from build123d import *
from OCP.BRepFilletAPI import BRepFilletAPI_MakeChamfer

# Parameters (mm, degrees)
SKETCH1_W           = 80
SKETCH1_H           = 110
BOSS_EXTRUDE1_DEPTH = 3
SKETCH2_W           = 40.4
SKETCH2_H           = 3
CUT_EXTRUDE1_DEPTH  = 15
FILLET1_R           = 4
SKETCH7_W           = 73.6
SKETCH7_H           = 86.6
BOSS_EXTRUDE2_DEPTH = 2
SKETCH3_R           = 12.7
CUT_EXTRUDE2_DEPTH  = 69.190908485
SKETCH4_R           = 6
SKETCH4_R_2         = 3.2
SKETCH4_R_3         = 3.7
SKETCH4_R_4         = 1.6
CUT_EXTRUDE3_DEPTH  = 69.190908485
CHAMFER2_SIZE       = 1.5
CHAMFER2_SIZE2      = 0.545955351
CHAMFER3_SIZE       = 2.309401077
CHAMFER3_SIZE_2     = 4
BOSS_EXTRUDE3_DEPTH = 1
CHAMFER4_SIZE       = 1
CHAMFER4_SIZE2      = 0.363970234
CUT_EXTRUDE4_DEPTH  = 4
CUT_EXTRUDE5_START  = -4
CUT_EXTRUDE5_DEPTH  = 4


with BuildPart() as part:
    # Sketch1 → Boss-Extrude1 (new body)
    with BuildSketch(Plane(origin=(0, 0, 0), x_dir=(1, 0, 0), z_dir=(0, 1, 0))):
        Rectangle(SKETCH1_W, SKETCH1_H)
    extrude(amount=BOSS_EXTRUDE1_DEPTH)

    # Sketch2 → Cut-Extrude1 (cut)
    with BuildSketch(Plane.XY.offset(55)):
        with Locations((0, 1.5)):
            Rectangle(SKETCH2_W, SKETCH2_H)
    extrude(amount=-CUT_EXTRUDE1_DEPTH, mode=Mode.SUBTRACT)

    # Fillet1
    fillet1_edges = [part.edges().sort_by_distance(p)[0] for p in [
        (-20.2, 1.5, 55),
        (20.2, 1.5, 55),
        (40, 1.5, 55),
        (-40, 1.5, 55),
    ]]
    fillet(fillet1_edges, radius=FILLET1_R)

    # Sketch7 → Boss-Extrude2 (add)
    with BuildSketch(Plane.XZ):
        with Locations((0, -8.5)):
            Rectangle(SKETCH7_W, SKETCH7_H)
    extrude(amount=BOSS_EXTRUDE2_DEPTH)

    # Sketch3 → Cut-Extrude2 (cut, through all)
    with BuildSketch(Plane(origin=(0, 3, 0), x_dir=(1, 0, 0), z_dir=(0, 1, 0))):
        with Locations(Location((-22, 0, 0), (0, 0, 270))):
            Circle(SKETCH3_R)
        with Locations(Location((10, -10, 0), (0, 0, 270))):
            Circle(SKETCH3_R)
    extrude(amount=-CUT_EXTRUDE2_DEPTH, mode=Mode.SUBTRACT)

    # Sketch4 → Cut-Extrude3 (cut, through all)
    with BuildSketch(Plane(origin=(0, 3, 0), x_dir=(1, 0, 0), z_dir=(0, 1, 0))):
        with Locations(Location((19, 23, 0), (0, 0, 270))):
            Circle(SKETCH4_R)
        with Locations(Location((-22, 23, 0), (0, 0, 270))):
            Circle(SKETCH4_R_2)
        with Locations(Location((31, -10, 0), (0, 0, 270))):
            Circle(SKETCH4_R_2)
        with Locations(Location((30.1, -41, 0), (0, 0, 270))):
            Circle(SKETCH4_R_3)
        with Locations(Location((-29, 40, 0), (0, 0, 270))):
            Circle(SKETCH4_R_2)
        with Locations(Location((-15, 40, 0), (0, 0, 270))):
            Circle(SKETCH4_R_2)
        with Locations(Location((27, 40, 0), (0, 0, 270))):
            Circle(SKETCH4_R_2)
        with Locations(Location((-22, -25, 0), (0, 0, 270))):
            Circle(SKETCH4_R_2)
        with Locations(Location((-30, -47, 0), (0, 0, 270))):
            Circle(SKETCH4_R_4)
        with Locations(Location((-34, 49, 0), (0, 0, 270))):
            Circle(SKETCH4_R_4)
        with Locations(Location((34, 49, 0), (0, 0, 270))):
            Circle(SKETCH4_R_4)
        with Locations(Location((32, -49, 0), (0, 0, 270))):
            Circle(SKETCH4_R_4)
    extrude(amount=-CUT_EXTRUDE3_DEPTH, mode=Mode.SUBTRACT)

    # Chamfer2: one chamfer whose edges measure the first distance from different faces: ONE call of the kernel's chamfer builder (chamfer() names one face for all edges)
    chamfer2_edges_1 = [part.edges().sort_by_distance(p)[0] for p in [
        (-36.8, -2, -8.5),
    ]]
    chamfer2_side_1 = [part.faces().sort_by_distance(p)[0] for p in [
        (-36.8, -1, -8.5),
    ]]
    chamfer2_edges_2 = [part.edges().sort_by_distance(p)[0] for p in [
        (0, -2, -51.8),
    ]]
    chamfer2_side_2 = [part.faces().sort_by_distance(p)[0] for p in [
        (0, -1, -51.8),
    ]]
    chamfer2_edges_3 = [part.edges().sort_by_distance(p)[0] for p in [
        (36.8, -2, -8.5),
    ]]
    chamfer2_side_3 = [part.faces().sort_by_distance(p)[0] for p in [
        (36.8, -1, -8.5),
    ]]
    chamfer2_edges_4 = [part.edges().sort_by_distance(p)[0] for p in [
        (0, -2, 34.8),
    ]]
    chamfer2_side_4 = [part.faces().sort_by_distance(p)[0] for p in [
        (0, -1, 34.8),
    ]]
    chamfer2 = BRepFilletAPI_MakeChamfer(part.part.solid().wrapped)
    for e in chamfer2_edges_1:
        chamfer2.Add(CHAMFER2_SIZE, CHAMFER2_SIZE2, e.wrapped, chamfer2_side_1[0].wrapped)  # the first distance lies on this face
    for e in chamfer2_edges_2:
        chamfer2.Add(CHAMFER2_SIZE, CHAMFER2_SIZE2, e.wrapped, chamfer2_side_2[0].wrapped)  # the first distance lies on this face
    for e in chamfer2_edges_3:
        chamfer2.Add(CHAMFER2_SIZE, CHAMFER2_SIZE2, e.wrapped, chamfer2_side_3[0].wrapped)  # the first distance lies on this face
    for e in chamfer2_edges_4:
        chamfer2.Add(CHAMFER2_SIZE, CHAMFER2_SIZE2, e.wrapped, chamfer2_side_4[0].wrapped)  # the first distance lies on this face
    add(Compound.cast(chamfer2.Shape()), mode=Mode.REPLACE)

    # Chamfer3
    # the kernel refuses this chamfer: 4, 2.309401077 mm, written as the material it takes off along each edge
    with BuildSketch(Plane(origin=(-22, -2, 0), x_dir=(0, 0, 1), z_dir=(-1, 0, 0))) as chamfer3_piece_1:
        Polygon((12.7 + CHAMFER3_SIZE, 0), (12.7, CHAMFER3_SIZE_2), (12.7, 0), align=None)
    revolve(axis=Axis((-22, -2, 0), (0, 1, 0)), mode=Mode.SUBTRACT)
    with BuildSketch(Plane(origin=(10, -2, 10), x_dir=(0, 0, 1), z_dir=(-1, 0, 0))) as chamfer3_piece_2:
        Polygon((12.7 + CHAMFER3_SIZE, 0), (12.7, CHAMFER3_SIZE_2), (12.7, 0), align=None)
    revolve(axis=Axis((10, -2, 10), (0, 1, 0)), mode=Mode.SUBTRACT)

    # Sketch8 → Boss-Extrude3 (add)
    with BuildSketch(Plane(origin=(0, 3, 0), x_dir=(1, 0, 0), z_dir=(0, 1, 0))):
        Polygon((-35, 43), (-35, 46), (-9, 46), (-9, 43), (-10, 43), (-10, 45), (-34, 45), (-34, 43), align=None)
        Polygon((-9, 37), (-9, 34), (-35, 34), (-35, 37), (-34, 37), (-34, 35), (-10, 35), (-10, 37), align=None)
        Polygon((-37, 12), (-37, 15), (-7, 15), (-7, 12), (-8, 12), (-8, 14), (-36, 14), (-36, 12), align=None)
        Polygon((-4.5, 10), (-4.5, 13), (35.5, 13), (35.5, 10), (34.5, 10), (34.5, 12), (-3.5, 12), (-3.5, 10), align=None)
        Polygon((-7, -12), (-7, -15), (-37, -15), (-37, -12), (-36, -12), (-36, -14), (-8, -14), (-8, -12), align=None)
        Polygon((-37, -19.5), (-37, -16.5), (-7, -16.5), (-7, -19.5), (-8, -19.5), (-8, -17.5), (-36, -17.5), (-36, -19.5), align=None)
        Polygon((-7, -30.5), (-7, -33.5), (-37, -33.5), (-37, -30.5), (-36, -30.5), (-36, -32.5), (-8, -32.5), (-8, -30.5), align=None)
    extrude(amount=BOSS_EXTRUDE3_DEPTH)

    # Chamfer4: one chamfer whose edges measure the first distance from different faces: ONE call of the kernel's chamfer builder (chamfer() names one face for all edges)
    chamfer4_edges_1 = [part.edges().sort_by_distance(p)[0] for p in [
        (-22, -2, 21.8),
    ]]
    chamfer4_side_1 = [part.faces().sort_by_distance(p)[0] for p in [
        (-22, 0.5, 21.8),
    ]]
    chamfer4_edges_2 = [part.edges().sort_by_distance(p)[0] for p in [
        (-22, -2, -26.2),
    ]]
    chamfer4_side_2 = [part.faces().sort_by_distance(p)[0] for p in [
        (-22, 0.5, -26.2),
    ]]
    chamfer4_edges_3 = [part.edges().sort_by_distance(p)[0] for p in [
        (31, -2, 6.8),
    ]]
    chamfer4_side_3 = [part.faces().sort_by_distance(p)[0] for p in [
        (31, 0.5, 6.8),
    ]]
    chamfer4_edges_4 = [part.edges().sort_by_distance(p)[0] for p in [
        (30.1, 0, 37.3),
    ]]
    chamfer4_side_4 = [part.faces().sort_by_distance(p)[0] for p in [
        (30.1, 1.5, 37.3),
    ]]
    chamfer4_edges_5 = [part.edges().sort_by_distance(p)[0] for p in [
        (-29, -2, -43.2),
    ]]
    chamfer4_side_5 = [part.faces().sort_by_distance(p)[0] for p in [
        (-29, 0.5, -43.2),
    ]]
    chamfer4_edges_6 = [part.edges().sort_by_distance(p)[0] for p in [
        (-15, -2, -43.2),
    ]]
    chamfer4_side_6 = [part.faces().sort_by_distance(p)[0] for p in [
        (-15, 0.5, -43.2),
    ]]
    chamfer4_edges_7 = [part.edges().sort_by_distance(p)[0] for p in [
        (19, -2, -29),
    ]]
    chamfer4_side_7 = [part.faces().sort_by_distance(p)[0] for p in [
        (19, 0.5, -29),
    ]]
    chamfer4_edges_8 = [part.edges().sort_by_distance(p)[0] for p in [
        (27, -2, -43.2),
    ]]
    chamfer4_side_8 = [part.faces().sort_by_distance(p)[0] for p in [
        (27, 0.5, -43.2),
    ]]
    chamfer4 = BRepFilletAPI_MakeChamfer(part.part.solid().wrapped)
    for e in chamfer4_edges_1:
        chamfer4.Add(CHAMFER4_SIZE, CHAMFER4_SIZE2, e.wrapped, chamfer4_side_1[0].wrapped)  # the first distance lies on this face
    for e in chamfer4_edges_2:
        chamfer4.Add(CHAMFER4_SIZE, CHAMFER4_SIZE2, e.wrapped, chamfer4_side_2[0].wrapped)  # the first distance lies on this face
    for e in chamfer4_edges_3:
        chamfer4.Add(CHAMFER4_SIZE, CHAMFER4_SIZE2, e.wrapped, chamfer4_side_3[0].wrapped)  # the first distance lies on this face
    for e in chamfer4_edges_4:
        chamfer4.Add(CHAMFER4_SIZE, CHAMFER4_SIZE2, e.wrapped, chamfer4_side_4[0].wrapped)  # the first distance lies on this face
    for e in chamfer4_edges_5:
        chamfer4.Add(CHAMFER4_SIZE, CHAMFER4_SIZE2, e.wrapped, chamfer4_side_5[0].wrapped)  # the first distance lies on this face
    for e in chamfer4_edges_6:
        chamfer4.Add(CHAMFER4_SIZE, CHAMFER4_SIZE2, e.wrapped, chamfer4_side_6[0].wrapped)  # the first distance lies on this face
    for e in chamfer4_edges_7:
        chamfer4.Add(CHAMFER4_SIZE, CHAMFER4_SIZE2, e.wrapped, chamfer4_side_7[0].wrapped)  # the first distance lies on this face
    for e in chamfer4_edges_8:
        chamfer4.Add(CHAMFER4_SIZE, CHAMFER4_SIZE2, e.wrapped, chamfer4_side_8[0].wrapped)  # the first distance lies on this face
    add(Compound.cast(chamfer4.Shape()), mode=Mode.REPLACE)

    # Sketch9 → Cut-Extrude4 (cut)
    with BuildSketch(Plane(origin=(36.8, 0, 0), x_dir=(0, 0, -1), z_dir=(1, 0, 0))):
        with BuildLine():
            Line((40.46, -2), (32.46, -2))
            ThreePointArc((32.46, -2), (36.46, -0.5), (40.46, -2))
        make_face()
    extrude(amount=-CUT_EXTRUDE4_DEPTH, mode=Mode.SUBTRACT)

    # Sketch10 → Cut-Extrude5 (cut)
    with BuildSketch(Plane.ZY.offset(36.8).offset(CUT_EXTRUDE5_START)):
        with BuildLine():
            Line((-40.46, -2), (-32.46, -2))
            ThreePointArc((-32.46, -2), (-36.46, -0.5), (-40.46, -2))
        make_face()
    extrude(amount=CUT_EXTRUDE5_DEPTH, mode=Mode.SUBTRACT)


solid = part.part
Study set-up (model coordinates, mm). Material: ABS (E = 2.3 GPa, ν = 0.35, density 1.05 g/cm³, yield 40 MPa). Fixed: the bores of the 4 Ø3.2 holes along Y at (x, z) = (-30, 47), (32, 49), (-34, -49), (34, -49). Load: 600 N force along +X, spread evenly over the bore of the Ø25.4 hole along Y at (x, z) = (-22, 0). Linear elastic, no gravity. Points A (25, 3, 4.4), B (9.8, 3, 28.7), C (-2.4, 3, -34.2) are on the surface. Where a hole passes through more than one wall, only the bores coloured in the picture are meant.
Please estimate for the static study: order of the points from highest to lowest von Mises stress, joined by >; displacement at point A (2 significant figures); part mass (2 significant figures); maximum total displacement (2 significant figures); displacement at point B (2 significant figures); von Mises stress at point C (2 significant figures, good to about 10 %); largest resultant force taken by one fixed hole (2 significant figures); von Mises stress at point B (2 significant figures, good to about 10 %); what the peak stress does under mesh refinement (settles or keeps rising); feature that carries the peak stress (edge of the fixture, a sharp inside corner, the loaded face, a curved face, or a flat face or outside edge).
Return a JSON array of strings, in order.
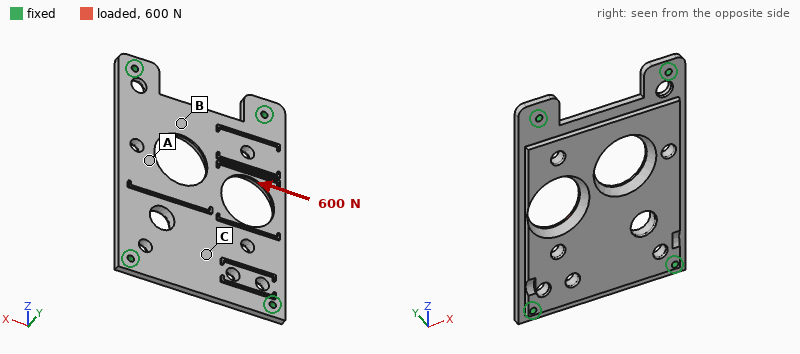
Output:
["B > C > A", "0.15 mm", "31 g", "0.63 mm", "0.14 mm", "3.2 MPa", "230 N", "5.9 MPa", "keeps rising", "edge of the fixture"]
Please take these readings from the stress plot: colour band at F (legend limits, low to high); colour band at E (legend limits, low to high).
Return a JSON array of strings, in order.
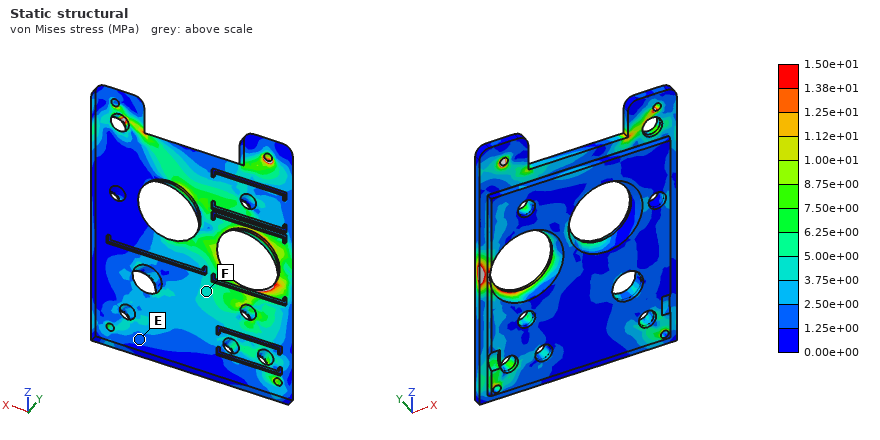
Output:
["3.75e+00 to 5.00e+00 MPa", "1.25e+00 to 2.50e+00 MPa"]
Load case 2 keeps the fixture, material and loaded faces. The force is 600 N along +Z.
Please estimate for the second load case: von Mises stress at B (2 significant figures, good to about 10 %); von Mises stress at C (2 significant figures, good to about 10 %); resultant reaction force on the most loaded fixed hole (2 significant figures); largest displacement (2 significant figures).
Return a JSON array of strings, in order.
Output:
["1.7 MPa", "0.91 MPa", "240 N", "0.19 mm"]
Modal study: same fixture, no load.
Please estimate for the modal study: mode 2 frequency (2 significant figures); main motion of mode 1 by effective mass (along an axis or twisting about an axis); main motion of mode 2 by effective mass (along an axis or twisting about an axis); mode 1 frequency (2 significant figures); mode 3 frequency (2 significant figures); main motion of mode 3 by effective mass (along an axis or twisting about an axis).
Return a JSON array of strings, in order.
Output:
["810 Hz", "along Y", "twisting about Z", "480 Hz", "1200 Hz", "twisting about X"]
